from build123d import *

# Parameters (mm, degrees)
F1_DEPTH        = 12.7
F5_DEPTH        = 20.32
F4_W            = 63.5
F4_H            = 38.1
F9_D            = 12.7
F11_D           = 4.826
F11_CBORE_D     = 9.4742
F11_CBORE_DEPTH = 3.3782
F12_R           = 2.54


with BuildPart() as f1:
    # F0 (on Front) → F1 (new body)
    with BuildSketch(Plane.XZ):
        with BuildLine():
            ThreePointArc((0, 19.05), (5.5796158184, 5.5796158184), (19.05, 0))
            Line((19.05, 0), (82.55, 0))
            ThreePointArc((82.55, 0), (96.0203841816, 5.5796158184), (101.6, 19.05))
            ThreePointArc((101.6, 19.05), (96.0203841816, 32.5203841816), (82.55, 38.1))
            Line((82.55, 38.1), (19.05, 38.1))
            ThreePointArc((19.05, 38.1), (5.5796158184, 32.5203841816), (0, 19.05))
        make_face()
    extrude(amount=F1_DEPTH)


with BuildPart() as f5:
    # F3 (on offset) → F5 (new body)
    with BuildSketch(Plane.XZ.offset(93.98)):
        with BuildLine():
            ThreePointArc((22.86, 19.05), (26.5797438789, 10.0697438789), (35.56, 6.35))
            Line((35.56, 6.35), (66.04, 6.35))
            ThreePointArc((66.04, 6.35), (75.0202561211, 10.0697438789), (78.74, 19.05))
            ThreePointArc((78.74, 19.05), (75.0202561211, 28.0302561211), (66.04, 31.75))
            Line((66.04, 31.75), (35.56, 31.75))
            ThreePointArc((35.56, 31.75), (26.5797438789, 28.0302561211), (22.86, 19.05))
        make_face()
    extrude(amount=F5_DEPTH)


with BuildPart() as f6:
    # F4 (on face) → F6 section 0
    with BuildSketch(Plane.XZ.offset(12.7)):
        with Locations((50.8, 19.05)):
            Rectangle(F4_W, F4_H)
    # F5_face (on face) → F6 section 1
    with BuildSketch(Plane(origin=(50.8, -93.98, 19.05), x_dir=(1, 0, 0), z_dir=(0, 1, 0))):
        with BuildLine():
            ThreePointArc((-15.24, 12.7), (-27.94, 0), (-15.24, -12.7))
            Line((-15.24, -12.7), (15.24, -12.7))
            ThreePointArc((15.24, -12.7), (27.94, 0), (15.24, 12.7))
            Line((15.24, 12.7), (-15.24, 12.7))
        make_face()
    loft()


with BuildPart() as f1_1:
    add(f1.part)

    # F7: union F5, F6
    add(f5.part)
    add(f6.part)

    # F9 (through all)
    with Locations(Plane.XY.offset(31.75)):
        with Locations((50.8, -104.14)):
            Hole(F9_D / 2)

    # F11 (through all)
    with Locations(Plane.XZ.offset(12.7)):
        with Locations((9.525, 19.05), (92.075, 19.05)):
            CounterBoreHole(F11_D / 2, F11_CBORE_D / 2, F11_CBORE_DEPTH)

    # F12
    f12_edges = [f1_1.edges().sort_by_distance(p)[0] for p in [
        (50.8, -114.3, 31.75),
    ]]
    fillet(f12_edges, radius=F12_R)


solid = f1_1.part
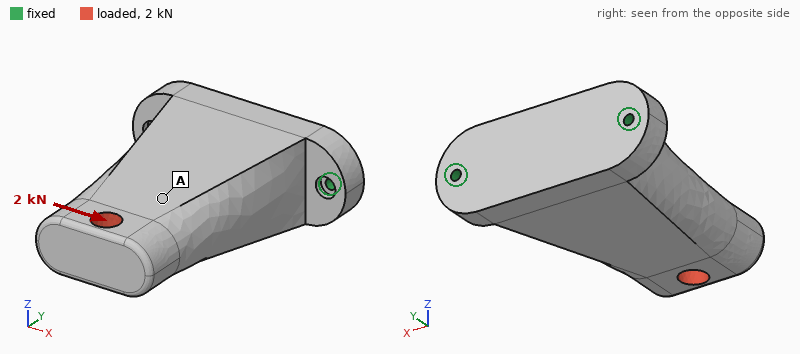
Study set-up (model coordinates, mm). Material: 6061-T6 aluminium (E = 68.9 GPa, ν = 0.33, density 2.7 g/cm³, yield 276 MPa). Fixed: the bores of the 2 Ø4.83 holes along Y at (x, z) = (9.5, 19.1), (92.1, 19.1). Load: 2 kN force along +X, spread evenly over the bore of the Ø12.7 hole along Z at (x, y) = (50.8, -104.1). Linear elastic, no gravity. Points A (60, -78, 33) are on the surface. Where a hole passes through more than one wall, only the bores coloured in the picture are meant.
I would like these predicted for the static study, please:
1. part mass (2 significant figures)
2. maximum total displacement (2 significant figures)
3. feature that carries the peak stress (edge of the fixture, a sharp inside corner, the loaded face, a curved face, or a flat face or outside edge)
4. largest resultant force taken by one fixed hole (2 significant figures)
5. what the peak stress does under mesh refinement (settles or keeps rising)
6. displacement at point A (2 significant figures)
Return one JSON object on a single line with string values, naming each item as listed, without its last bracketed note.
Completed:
{"part mass": "580 g", "maximum total displacement": "50 µm", "feature that carries the peak stress": "edge of the fixture", "largest resultant force taken by one fixed hole": "2.8 kN", "what the peak stress does under mesh refinement": "keeps rising", "displacement at point A": "28 µm"}
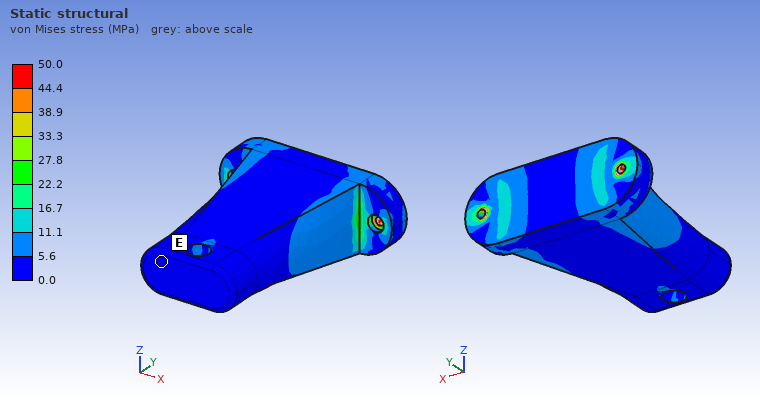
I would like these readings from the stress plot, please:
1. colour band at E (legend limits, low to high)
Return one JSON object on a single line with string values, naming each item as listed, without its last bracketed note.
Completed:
{"colour band at E": "0.0 to 5.6 MPa"}
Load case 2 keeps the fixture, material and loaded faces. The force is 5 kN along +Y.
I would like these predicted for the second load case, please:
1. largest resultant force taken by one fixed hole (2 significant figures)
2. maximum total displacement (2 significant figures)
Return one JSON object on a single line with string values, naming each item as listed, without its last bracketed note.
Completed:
{"largest resultant force taken by one fixed hole": "2.8 kN", "maximum total displacement": "18 µm"}
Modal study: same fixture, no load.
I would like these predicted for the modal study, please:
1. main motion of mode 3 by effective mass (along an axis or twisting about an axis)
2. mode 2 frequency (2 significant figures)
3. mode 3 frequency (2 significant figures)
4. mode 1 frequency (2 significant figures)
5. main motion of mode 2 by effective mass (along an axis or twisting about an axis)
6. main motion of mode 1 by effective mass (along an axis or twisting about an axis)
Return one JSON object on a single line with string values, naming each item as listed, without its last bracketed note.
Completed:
{"main motion of mode 3 by effective mass": "along Y", "mode 2 frequency": "2800 Hz", "mode 3 frequency": "4600 Hz", "mode 1 frequency": "730 Hz", "main motion of mode 2 by effective mass": "along X", "main motion of mode 1 by effective mass": "along Z"}
